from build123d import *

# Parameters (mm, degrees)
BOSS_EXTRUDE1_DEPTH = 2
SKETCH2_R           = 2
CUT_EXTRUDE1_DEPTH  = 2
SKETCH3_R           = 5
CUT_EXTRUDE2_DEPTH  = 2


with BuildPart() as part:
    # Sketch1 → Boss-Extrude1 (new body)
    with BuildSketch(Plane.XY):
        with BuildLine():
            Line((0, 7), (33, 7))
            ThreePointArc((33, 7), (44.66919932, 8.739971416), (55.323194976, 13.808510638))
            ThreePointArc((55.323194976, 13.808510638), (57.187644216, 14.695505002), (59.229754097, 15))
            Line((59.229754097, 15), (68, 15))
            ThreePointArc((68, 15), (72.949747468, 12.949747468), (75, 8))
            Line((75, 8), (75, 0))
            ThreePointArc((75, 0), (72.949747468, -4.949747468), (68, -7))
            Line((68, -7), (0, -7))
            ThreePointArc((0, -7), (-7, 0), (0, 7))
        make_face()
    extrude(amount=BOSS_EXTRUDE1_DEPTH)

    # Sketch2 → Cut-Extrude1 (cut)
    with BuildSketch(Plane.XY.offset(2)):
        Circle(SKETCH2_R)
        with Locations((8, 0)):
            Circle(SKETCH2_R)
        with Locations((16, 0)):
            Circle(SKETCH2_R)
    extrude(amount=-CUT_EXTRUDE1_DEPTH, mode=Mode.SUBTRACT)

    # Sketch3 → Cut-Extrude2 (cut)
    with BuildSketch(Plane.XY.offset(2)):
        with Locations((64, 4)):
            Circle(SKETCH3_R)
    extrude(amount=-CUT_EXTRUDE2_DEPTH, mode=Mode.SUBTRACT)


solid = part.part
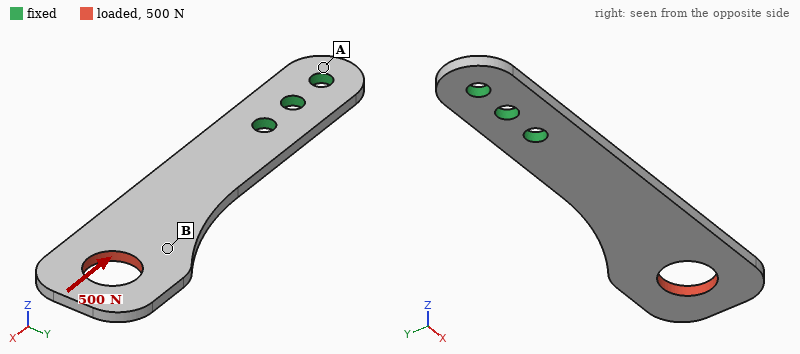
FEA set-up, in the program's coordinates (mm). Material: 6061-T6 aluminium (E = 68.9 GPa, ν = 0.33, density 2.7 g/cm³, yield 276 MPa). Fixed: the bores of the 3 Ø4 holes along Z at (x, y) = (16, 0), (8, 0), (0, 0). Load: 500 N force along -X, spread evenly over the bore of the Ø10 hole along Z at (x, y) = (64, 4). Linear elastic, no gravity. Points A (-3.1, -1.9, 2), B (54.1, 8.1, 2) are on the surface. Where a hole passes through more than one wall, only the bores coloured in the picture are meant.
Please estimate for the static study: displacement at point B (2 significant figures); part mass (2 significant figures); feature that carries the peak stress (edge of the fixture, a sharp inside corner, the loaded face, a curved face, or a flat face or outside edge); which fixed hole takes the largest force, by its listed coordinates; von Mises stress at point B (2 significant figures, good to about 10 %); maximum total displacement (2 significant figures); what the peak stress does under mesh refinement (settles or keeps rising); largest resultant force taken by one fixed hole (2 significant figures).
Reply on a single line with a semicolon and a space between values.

0.061 mm; 6.4 g; edge of the fixture; (16, 0); 18 MPa; 0.11 mm; keeps rising; 420 N
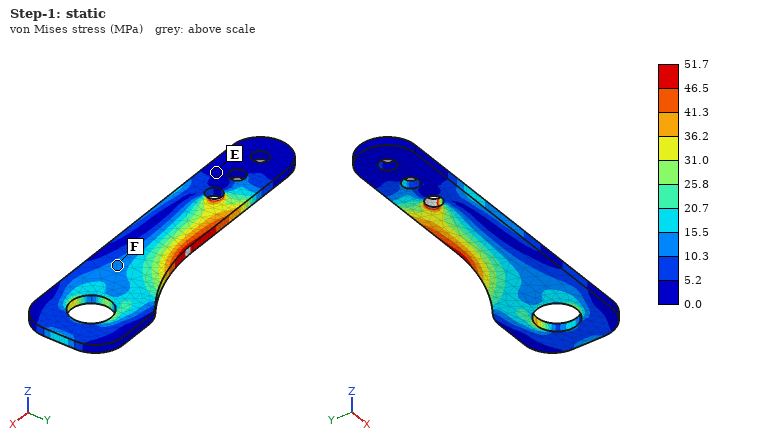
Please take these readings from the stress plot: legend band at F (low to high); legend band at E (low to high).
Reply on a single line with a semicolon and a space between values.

10.3 to 15.5 MPa; 0.0 to 5.2 MPa
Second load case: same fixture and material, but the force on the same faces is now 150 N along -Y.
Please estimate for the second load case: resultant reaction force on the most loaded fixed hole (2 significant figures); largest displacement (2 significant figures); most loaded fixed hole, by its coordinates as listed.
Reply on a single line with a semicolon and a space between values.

510 N; 0.30 mm; (16, 0)
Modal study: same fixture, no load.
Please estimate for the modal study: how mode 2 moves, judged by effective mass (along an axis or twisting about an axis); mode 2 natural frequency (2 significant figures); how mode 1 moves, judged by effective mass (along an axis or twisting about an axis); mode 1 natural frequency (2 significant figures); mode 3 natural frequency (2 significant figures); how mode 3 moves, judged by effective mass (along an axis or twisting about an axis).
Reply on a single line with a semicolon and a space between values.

twisting about X; 2300 Hz; along Z; 450 Hz; 2500 Hz; along Y
